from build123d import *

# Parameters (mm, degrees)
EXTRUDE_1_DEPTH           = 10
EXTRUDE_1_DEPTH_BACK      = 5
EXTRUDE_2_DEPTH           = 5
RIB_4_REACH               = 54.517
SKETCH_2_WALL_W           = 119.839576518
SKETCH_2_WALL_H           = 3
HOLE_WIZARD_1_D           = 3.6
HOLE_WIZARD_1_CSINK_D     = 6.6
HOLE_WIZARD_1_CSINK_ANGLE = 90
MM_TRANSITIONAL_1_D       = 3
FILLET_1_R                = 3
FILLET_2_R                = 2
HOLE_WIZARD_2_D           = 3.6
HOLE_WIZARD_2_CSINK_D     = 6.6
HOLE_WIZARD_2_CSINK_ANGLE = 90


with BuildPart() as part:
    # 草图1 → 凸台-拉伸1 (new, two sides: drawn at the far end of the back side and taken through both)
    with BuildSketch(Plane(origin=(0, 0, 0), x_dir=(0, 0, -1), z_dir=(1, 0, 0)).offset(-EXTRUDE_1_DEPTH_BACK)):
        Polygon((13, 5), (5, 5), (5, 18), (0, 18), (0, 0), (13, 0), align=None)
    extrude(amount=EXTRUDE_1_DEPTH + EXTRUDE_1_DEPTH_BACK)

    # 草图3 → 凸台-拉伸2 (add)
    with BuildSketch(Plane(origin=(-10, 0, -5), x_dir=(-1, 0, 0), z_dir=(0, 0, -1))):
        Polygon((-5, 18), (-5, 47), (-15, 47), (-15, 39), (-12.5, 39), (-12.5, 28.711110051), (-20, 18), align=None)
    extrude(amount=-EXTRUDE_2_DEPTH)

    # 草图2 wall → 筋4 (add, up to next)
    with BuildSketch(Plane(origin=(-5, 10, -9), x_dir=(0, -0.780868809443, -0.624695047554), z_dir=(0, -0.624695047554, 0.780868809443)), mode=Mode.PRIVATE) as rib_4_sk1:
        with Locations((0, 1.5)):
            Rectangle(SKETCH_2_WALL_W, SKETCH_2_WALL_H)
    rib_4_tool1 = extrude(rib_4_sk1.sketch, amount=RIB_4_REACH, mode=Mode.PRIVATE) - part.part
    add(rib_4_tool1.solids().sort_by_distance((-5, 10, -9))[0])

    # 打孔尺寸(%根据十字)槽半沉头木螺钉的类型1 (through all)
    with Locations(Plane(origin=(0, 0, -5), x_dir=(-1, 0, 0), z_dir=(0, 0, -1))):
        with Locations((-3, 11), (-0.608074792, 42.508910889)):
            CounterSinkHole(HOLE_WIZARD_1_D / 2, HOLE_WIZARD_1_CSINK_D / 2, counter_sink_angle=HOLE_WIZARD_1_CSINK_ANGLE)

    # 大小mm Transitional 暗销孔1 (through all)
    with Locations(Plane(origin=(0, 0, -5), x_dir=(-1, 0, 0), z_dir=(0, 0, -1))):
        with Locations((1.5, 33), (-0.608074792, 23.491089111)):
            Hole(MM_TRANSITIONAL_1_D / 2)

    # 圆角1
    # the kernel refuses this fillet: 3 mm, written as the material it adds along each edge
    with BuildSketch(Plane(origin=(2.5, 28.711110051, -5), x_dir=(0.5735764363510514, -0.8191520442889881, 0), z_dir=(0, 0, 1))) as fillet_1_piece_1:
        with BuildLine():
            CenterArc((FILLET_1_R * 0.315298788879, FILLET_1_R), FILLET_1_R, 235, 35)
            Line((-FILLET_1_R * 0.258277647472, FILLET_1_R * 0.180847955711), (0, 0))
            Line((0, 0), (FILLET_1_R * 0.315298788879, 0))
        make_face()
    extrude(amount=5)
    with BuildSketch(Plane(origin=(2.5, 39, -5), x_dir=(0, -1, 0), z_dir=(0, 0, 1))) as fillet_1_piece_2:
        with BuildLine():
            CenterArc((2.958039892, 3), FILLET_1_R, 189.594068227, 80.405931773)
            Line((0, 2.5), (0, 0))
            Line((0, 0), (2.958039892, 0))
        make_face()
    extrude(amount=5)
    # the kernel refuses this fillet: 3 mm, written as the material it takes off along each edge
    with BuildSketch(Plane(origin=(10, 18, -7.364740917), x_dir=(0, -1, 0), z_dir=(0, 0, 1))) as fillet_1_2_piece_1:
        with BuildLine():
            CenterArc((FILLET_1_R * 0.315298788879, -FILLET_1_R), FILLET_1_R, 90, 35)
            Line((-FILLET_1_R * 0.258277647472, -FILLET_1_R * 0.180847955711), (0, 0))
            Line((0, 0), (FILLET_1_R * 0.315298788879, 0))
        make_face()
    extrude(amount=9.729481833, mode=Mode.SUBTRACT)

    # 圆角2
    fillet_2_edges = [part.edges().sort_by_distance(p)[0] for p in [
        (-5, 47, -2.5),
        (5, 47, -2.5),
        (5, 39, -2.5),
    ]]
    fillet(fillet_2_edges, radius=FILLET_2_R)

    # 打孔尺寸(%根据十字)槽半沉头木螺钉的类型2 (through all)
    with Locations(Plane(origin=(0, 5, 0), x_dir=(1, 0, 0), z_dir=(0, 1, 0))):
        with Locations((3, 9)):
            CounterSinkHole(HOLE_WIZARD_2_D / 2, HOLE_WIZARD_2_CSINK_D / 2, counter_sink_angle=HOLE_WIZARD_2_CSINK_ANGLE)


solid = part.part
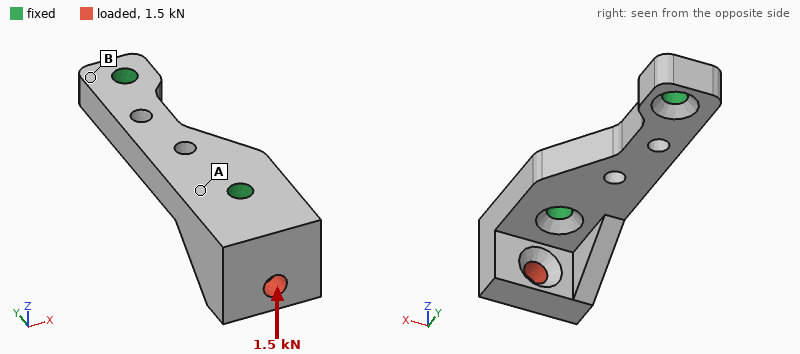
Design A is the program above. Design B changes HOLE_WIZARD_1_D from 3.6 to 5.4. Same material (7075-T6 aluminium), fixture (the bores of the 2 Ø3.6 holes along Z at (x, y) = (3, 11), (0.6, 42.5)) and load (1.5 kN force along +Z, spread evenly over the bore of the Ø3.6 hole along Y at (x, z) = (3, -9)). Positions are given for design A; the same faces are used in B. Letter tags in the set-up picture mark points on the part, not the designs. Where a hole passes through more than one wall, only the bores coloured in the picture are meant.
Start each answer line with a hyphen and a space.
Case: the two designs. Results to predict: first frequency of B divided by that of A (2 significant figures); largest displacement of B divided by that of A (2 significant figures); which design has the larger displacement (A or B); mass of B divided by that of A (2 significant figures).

- 1.4
- 0.58
- A
- 0.97
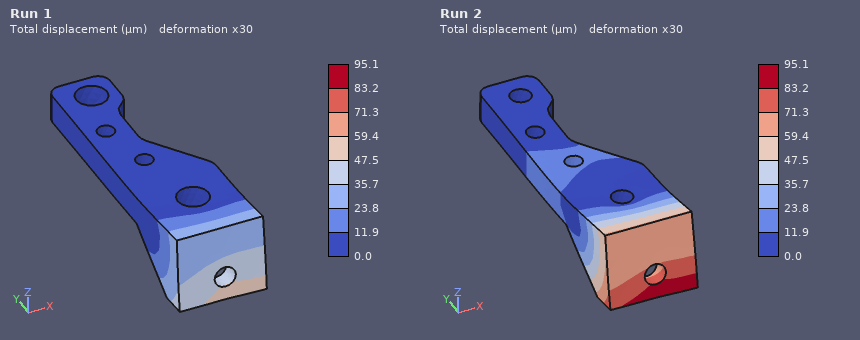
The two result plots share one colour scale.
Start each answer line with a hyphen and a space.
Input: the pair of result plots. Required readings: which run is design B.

- Run 1
